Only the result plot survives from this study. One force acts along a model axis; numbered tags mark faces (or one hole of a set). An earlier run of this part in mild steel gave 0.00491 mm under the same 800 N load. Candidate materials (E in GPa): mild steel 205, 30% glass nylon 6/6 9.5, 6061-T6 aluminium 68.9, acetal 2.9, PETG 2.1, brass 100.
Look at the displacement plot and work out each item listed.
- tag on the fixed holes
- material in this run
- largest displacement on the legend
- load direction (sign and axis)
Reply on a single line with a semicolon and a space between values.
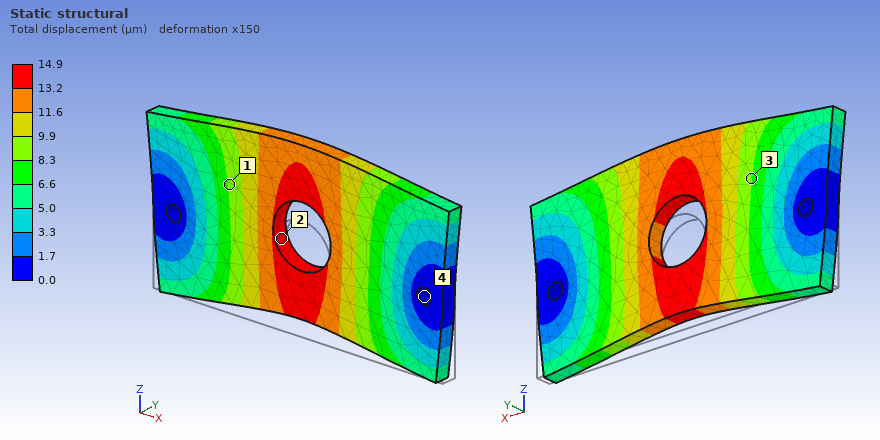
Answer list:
4; 6061-T6 aluminium; 14.9 µm; +Z
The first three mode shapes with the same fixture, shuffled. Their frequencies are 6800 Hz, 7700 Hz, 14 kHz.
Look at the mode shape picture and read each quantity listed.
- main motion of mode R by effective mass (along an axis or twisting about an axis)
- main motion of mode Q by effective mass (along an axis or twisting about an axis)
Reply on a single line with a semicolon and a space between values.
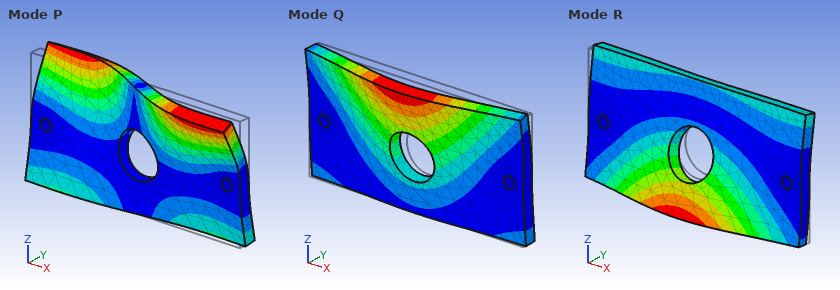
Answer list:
along Y; along Y
